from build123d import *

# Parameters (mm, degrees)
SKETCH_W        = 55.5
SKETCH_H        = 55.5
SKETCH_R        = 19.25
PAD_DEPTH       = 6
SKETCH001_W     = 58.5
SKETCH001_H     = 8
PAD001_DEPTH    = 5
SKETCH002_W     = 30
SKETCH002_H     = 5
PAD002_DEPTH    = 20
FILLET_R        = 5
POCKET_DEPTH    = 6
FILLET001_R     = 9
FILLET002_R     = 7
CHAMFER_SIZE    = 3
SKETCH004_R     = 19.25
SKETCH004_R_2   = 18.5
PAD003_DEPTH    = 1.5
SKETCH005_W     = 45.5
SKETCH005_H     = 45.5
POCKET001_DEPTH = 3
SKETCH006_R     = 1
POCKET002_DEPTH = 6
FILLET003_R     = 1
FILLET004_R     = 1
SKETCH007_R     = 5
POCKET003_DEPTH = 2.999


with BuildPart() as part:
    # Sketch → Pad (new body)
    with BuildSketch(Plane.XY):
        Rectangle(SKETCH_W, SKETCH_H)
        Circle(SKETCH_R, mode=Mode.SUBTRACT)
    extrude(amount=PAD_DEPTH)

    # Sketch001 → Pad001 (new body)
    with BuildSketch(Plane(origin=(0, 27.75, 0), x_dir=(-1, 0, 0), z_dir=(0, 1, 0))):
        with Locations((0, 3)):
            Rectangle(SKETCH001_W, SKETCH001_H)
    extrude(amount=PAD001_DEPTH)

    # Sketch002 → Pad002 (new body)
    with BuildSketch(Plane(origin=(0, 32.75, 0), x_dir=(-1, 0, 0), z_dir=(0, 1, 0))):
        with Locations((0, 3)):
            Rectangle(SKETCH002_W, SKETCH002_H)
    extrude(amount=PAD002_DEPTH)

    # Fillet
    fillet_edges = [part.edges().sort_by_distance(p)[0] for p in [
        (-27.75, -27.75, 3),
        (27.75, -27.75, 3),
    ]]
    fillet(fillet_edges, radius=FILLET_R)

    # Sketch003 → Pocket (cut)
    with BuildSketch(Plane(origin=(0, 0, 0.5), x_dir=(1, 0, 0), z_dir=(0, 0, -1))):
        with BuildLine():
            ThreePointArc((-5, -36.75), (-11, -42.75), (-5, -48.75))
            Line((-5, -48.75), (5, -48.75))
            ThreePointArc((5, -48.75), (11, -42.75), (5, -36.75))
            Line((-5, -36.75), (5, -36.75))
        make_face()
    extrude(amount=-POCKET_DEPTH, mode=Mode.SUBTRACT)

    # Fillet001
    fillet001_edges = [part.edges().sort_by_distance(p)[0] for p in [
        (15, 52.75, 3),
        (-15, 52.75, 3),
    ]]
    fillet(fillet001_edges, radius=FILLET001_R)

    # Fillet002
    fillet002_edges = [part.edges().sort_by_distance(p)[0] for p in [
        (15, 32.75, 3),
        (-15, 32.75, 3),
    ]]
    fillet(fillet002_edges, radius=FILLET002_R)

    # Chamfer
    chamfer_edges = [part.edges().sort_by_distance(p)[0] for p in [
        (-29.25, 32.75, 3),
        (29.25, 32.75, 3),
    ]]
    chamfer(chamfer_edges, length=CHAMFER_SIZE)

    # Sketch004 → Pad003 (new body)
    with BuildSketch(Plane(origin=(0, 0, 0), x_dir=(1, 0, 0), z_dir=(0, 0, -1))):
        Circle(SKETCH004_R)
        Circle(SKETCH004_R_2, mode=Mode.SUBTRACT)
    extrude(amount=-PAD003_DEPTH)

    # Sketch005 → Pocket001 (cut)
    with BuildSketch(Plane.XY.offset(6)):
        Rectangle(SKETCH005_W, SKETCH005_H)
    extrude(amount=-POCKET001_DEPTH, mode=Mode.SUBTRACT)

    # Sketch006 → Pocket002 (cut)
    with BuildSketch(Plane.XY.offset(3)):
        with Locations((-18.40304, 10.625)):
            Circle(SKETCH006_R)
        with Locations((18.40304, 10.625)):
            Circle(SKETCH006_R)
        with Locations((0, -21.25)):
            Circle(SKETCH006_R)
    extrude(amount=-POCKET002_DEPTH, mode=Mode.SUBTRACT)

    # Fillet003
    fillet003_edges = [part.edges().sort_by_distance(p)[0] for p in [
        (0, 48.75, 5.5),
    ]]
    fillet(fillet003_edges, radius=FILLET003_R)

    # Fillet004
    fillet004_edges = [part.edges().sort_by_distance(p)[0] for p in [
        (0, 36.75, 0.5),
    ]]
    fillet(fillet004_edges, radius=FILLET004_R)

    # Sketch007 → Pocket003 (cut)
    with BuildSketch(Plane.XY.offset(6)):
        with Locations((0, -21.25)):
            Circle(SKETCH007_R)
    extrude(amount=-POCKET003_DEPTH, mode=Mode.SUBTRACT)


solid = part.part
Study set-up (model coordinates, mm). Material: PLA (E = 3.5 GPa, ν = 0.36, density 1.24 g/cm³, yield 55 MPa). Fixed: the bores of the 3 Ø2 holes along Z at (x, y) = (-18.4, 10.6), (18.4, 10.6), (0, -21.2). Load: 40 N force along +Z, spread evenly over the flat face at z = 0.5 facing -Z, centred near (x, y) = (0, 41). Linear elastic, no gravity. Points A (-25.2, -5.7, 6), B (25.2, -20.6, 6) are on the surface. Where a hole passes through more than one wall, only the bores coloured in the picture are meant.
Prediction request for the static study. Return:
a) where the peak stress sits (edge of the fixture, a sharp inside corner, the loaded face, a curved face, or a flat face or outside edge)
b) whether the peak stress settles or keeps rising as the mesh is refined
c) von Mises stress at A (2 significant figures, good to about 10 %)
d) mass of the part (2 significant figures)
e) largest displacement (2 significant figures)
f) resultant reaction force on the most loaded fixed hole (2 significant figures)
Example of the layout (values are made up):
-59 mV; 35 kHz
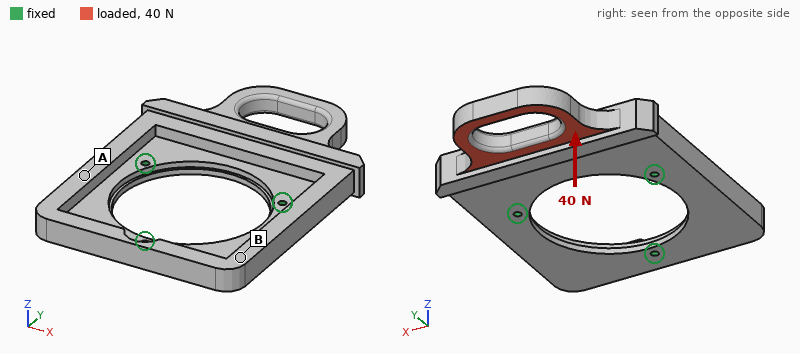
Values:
edge of the fixture; keeps rising; 3.7 MPa; 16 g; 1.1 mm; 31 N
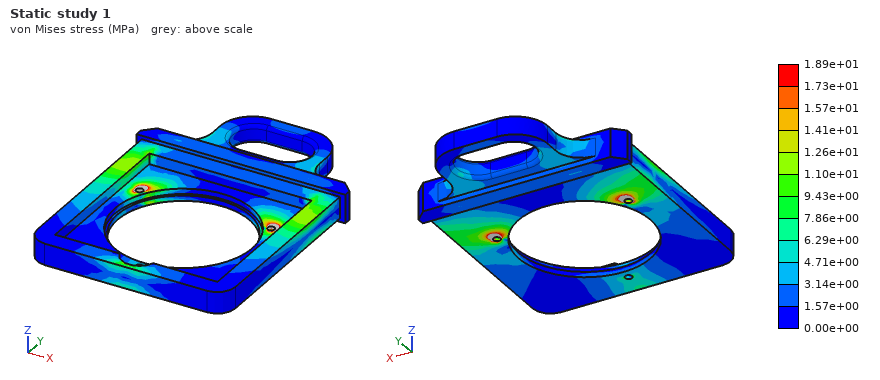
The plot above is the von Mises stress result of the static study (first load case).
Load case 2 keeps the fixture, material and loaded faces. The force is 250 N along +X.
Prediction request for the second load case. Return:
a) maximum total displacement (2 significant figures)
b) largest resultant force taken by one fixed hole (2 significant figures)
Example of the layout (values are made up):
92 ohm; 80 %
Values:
0.27 mm; 220 N
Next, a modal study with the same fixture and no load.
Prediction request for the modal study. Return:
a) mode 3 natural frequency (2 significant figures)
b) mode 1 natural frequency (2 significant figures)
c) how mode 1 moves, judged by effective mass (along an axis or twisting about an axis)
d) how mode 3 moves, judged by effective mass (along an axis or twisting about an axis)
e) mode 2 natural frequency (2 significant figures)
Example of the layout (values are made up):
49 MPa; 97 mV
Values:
1600 Hz; 610 Hz; along Z; along Z; 1100 Hz
